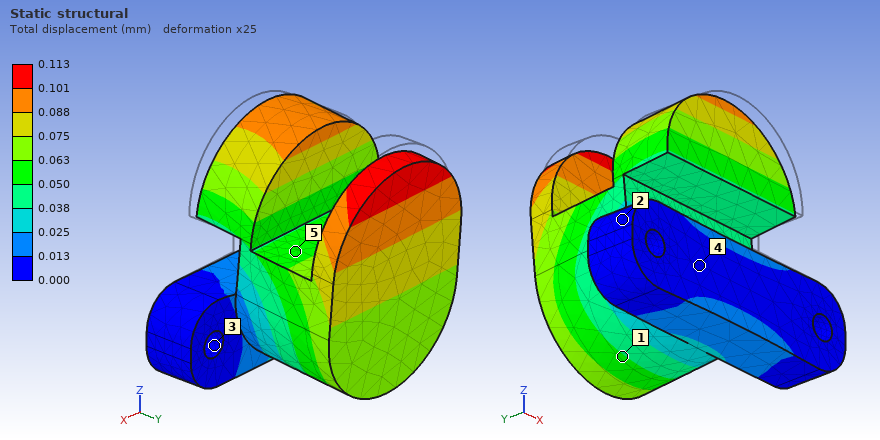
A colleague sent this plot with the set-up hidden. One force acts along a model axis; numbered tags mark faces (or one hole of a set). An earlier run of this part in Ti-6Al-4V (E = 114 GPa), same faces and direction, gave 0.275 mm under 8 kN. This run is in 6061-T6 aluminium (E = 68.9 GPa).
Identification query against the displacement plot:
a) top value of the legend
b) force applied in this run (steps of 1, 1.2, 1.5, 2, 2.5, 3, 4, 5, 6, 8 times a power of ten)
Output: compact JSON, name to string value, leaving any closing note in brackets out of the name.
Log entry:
{"top value of the legend": "0.113 mm", "force applied in this run": "2 kN"}
